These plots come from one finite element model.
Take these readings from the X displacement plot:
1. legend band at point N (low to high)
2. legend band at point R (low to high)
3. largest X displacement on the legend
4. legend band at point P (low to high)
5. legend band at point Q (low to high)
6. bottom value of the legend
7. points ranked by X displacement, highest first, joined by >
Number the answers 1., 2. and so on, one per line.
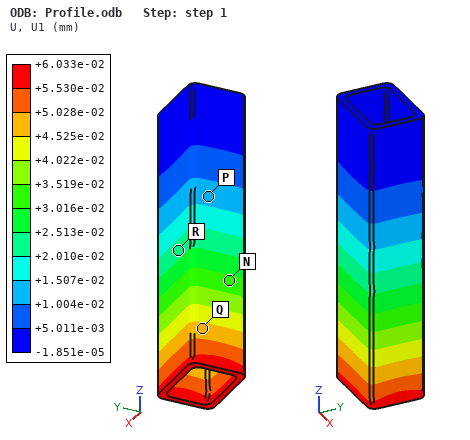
1. +3.016e-02 to +3.519e-02 mm
2. +2.010e-02 to +2.513e-02 mm
3. +6.033e-02 mm
4. +1.004e-02 to +1.507e-02 mm
5. +4.525e-02 to +5.028e-02 mm
6. -1.851e-05 mm
7. Q > N > R > P
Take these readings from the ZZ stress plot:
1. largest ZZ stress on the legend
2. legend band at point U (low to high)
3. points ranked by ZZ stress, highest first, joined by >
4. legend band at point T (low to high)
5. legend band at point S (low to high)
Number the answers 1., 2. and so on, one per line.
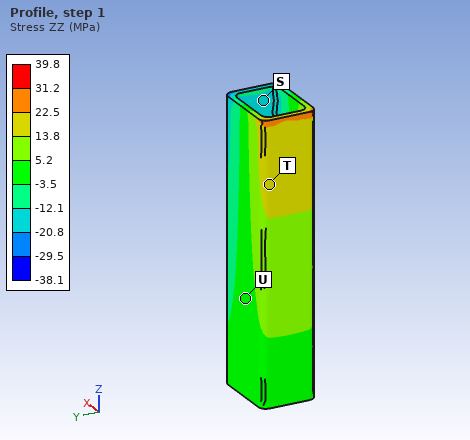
1. 39.8 MPa
2. -3.5 to 5.2 MPa
3. T > U > S
4. 13.8 to 22.5 MPa
5. -20.8 to -12.1 MPa
